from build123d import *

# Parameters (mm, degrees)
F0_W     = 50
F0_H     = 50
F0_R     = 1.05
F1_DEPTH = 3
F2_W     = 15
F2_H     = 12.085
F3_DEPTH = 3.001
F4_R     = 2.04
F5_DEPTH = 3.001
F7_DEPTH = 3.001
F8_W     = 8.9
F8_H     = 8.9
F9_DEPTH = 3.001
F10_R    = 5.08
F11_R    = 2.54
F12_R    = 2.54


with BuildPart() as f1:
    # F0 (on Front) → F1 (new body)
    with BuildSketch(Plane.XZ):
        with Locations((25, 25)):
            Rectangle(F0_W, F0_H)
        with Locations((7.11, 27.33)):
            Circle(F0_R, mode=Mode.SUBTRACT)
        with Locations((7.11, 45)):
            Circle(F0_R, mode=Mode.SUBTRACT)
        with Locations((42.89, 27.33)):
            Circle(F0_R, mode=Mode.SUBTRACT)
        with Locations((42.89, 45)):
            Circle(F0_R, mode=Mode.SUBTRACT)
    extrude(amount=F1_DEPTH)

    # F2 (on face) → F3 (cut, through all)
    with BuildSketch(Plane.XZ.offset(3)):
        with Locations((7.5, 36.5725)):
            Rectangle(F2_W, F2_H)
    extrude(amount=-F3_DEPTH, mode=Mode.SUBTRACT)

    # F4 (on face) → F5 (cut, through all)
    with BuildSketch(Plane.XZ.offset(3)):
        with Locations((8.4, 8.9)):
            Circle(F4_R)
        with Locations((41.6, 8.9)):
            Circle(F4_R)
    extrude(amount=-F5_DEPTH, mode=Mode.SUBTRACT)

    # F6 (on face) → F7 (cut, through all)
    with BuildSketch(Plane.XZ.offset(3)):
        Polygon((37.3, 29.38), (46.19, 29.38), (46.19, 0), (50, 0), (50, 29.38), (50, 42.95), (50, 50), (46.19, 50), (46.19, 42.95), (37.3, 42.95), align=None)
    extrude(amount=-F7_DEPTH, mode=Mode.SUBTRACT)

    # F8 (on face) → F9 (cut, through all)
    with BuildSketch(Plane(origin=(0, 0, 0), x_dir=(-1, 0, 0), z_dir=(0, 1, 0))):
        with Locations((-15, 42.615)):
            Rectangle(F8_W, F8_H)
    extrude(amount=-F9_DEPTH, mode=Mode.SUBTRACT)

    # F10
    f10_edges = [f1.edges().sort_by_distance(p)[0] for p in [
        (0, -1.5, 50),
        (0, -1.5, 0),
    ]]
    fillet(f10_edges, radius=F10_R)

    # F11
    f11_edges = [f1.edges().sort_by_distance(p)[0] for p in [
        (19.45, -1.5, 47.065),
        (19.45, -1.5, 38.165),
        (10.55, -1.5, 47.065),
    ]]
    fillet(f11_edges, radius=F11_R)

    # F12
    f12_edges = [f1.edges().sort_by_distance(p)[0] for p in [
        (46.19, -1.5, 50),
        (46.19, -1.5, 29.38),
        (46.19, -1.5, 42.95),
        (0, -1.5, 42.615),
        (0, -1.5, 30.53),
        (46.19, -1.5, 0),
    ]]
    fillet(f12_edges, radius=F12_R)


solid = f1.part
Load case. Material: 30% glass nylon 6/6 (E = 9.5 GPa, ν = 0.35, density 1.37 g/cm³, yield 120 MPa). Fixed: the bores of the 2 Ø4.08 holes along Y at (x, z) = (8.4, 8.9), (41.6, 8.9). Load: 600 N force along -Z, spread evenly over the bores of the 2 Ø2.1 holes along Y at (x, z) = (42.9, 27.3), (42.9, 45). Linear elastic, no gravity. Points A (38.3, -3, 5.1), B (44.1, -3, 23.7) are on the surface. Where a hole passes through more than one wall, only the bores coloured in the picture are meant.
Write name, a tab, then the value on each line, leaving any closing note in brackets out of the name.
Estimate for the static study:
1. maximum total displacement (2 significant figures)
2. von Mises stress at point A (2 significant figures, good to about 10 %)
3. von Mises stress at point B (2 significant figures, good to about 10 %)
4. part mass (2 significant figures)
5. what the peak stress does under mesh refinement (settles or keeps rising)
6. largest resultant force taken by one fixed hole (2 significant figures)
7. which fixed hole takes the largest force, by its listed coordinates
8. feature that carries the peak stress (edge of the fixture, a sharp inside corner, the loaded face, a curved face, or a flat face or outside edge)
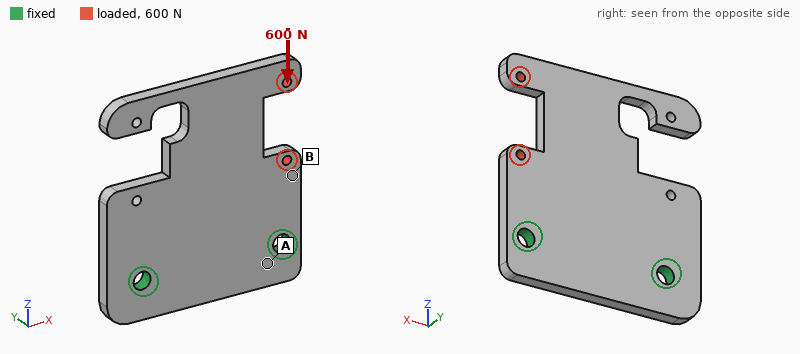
maximum total displacement	0.33 mm
von Mises stress at point A	6.8 MPa
von Mises stress at point B	17 MPa
part mass	7.8 g
what the peak stress does under mesh refinement	keeps rising
largest resultant force taken by one fixed hole	620 N
which fixed hole takes the largest force, by its listed coordinates	(41.6, 8.9)
feature that carries the peak stress	a sharp inside corner
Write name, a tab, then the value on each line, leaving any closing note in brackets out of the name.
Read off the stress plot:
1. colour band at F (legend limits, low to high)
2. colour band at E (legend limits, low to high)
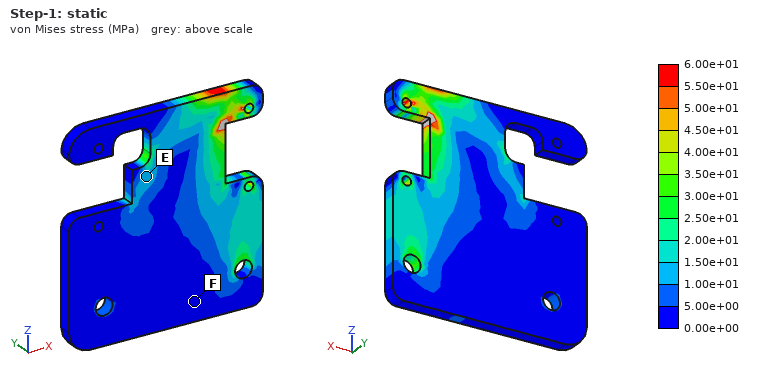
colour band at F	0.00e+00 to 5.00e+00 MPa
colour band at E	1.00e+01 to 1.50e+01 MPa
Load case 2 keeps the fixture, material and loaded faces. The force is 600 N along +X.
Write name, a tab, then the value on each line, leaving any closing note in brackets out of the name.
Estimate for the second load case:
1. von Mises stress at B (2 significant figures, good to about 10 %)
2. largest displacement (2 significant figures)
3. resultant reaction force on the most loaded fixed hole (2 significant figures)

von Mises stress at B	7.4 MPa
largest displacement	0.16 mm
resultant reaction force on the most loaded fixed hole	570 N
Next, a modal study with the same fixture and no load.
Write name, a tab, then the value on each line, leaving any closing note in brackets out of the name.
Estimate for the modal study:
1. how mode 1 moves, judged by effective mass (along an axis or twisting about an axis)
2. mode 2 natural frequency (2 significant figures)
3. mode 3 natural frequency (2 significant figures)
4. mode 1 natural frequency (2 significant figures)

how mode 1 moves, judged by effective mass	along Y
mode 2 natural frequency	1400 Hz
mode 3 natural frequency	2200 Hz
mode 1 natural frequency	770 Hz
